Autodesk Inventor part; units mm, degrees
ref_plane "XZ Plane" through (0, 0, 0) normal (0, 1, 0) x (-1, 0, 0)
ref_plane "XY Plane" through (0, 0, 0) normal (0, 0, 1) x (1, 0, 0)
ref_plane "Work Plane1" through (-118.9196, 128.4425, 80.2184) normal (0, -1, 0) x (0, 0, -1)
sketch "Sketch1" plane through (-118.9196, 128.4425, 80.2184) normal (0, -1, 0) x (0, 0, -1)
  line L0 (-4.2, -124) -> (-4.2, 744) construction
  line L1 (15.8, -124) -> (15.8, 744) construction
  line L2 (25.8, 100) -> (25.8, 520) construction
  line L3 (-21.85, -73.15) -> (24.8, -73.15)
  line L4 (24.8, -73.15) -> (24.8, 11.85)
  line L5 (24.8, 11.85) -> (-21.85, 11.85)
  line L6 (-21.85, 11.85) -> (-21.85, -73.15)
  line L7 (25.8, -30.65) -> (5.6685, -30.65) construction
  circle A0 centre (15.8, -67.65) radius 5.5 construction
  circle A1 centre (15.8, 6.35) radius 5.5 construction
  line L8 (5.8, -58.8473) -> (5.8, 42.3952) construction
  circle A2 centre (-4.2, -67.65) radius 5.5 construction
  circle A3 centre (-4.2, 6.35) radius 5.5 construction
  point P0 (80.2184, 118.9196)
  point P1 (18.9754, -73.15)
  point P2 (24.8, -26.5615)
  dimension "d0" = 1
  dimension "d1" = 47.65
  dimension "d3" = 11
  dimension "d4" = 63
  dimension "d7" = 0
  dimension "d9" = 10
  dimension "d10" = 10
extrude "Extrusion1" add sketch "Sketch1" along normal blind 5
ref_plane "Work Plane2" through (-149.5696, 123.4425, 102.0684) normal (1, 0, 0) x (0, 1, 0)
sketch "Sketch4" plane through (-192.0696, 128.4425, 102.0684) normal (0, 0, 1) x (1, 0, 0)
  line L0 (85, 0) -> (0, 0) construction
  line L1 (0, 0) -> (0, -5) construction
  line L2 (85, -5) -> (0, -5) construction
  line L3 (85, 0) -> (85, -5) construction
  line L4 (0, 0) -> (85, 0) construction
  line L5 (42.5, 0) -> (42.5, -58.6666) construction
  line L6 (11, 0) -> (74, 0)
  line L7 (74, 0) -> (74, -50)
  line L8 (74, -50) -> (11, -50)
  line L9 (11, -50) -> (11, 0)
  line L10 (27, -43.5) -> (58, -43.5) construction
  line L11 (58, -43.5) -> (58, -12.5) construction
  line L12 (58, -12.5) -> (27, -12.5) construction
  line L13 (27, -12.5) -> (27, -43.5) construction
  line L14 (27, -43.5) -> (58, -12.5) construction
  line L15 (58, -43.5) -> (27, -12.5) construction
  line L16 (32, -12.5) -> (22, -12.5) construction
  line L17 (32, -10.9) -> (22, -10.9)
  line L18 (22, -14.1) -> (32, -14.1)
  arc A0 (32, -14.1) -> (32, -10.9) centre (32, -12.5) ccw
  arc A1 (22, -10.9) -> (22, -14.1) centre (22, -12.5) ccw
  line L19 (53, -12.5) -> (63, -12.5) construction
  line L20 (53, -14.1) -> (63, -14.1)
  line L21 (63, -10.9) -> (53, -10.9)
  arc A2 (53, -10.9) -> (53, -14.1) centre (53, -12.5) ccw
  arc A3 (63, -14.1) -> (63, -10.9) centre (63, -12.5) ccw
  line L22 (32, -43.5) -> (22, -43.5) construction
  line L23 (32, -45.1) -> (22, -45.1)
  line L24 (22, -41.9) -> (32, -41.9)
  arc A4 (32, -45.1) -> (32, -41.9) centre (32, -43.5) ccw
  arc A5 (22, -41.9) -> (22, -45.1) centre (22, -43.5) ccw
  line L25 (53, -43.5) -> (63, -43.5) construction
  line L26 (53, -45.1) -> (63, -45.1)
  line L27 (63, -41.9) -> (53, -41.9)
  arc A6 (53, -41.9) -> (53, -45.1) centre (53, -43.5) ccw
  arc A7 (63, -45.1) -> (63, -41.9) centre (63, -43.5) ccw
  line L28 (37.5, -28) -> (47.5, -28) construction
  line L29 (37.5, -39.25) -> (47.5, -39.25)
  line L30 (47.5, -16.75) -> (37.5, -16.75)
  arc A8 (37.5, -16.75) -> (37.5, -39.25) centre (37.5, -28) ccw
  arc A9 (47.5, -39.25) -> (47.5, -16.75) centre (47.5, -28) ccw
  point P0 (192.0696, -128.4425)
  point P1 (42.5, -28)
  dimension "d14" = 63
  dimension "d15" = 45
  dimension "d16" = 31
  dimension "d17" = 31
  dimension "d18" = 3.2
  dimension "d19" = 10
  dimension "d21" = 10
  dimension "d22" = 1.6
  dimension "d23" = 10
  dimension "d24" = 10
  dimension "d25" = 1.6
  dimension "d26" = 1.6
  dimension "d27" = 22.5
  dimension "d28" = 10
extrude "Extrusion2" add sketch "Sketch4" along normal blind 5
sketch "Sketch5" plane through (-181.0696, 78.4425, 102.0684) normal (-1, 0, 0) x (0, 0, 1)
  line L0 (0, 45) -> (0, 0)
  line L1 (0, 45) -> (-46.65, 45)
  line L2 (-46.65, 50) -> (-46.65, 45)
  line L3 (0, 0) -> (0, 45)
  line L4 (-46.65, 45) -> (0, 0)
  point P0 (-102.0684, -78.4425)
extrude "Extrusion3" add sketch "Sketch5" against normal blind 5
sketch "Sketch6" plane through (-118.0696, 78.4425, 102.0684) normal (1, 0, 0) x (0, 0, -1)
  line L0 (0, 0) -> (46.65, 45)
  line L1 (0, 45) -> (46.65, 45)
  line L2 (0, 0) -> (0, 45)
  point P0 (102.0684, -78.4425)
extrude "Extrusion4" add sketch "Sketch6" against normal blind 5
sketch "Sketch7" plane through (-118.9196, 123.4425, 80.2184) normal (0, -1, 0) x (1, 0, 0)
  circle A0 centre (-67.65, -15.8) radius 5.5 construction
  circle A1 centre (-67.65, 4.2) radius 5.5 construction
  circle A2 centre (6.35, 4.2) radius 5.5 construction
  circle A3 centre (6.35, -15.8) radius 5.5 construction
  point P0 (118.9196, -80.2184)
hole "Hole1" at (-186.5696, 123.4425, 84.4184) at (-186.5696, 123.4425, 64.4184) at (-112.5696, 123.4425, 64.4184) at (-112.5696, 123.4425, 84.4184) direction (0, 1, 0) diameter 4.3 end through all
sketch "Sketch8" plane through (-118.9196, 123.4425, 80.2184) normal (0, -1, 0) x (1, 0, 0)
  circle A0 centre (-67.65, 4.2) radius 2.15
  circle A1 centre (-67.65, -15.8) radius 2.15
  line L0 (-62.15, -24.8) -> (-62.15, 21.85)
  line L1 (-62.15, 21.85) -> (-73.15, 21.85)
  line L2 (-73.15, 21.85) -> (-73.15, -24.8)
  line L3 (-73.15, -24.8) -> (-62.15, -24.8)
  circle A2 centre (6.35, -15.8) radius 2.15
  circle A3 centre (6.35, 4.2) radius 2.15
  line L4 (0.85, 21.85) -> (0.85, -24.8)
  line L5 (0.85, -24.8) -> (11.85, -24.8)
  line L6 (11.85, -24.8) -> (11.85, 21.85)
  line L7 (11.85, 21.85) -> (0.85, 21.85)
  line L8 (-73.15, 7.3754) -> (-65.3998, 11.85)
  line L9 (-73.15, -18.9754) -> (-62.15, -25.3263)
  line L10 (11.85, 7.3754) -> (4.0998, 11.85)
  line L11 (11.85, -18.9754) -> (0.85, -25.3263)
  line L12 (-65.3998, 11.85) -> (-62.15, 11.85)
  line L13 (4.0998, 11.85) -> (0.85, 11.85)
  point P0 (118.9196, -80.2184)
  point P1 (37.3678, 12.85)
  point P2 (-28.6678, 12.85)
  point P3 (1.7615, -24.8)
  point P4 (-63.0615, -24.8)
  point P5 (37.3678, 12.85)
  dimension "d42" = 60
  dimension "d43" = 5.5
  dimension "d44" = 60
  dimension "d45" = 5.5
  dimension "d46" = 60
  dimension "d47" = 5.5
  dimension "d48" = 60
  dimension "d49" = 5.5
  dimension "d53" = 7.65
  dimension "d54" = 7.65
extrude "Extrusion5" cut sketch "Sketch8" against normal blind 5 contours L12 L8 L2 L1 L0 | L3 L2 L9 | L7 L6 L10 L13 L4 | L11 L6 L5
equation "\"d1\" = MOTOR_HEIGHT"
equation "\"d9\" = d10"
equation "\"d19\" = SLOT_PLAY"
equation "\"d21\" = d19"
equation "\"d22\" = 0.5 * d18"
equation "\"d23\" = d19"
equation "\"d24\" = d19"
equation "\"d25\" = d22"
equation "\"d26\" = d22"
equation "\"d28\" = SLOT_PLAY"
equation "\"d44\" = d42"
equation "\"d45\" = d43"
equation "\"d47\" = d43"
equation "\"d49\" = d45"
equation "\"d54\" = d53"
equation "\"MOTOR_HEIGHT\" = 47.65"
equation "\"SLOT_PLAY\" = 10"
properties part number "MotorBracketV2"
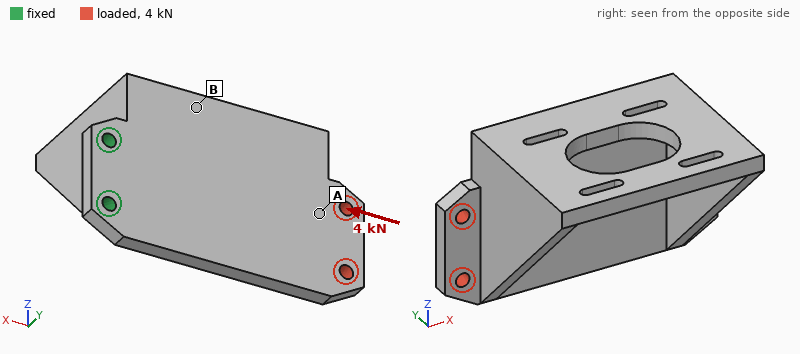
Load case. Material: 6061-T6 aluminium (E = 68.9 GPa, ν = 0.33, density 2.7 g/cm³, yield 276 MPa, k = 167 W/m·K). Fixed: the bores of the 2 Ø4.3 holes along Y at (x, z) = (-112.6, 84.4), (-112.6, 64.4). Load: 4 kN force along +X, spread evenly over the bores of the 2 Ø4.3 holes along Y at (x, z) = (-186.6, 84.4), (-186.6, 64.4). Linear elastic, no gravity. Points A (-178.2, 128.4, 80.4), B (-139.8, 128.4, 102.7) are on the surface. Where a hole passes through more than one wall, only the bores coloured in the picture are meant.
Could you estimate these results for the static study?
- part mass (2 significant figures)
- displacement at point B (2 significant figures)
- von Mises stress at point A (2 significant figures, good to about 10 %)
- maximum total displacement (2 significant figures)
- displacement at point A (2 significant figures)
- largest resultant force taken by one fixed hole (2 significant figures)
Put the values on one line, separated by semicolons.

110 g; 9.0 µm; 24 MPa; 35 µm; 24 µm; 2.0 kN
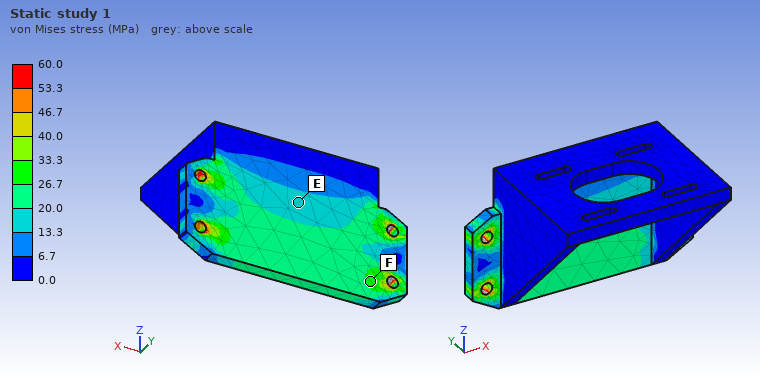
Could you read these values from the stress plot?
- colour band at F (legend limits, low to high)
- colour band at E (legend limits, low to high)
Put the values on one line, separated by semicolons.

26.7 to 33.3 MPa; 13.3 to 20.0 MPa
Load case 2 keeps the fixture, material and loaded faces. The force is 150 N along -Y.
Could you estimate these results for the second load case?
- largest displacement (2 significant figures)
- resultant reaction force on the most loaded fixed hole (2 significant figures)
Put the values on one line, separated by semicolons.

0.43 mm; 84 N
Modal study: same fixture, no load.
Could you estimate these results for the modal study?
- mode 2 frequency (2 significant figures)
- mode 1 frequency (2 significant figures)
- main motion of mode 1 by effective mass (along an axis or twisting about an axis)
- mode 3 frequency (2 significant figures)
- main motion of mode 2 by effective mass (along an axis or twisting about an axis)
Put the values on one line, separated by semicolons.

1400 Hz; 490 Hz; along Y; 2600 Hz; along Z
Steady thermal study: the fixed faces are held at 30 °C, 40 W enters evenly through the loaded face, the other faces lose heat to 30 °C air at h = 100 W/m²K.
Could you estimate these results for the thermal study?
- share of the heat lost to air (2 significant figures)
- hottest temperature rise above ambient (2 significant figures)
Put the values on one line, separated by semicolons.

65 %; 45 K
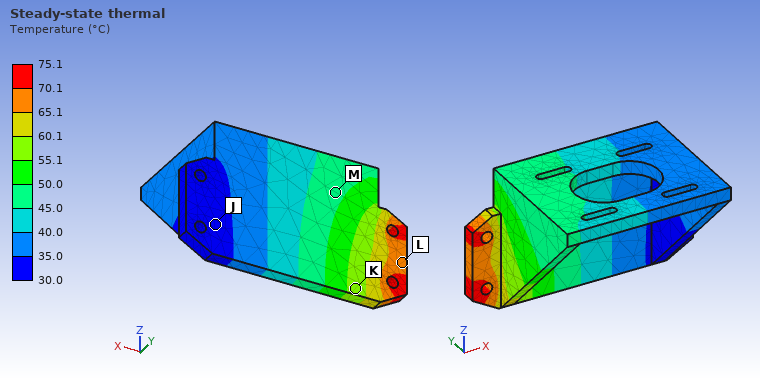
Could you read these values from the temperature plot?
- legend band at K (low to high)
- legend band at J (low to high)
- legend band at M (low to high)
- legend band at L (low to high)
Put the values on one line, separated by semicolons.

55.1 to 60.1 °C; 30.0 to 35.0 °C; 45.0 to 50.0 °C; 65.1 to 70.1 °C
